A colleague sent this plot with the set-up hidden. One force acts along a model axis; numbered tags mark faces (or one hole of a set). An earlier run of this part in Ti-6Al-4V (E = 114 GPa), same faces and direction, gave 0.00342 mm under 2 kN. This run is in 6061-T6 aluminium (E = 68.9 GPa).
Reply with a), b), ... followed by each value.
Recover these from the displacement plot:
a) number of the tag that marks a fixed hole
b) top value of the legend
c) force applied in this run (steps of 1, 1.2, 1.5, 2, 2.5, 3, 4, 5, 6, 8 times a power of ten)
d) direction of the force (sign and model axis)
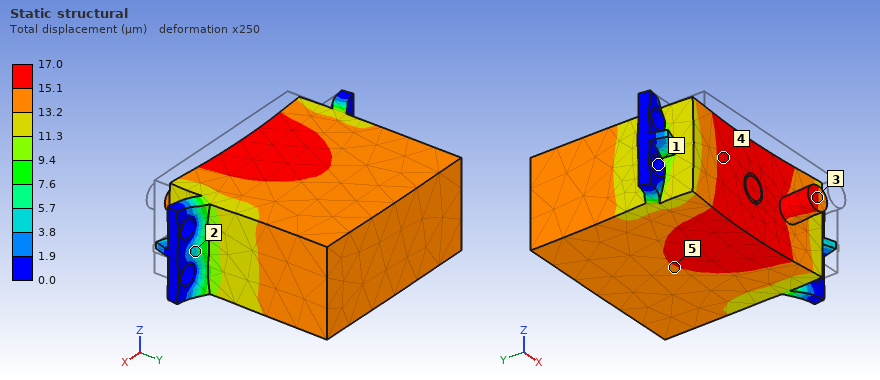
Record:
a) 1
b) 17.0 µm
c) 6 kN
d) +Y
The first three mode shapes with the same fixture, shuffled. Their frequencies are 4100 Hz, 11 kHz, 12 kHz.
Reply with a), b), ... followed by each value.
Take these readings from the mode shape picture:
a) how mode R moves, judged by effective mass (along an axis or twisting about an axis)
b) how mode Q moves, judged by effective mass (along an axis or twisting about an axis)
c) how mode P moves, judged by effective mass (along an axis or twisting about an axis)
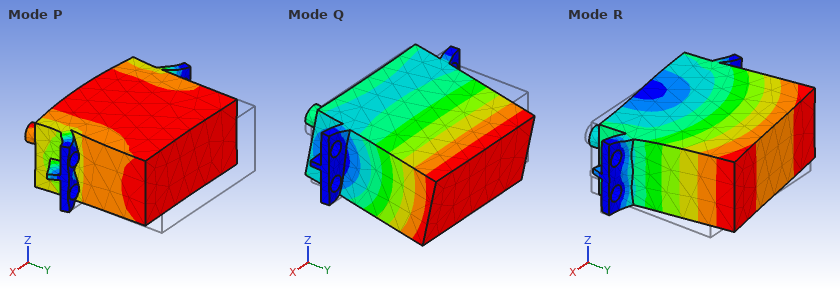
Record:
a) along X
b) along Z
c) along Y
